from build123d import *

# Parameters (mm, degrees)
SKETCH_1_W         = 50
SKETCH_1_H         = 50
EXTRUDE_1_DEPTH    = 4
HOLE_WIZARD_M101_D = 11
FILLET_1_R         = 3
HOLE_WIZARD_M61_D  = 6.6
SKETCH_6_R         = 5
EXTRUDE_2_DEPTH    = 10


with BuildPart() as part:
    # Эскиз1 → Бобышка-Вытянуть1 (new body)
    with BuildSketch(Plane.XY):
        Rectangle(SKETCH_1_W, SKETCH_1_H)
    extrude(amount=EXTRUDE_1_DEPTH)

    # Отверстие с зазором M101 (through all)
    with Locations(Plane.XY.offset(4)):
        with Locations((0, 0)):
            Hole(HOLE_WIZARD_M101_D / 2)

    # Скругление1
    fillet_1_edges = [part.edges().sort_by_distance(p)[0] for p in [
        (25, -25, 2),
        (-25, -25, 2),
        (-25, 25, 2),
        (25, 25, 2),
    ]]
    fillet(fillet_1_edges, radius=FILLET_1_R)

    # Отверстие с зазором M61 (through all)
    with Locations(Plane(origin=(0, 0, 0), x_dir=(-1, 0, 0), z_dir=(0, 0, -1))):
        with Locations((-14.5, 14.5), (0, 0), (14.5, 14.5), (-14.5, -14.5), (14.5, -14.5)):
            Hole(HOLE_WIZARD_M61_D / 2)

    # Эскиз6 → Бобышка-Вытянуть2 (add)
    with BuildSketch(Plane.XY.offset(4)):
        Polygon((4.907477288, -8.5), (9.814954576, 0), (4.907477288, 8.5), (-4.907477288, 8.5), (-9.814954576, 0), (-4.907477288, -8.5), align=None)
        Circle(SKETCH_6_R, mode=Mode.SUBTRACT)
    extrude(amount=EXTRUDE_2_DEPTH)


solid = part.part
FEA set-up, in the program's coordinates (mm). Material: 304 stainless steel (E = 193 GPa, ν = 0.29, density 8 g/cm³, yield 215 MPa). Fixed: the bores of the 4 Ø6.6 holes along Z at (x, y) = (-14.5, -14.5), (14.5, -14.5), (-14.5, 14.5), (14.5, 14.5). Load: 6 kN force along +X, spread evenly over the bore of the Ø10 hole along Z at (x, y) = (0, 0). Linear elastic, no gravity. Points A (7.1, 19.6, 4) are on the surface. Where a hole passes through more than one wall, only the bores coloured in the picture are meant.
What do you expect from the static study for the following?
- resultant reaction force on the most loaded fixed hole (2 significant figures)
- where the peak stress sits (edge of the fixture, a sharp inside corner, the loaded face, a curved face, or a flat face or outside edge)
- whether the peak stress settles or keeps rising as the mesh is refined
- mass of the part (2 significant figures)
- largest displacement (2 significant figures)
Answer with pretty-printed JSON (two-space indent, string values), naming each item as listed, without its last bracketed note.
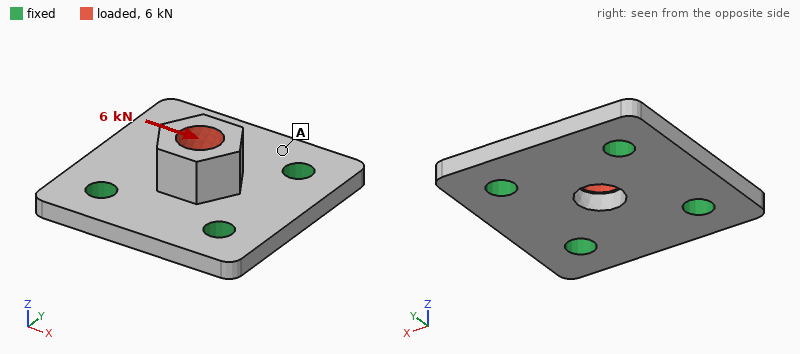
{
  "resultant reaction force on the most loaded fixed hole": "1.9 kN",
  "where the peak stress sits": "edge of the fixture",
  "whether the peak stress settles or keeps rising as the mesh is refined": "keeps rising",
  "mass of the part": "86 g",
  "largest displacement": "22 µm"
}
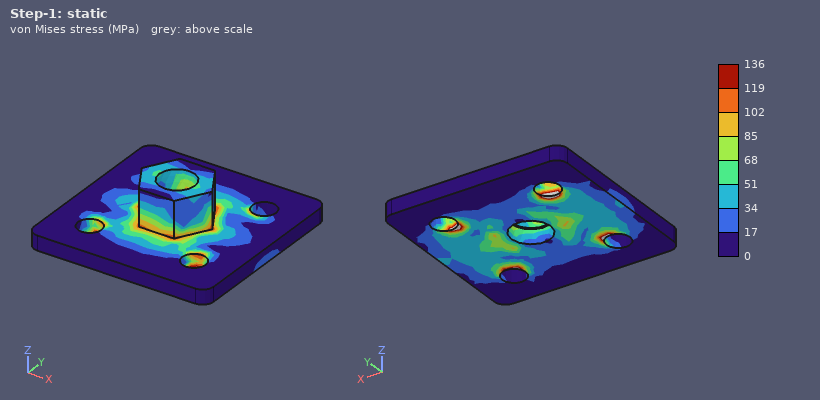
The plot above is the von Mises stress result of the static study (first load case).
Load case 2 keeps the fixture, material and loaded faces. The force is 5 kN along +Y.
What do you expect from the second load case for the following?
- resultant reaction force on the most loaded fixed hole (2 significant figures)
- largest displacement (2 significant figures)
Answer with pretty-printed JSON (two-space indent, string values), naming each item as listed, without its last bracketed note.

{
  "resultant reaction force on the most loaded fixed hole": "1.5 kN",
  "largest displacement": "18 µm"
}
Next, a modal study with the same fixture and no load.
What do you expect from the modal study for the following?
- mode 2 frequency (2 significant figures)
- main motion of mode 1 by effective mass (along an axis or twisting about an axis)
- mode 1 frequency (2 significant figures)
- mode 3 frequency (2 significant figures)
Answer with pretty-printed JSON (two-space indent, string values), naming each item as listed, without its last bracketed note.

{
  "mode 2 frequency": "22 kHz",
  "main motion of mode 1 by effective mass": "along Z",
  "mode 1 frequency": "19 kHz",
  "mode 3 frequency": "22 kHz"
}
